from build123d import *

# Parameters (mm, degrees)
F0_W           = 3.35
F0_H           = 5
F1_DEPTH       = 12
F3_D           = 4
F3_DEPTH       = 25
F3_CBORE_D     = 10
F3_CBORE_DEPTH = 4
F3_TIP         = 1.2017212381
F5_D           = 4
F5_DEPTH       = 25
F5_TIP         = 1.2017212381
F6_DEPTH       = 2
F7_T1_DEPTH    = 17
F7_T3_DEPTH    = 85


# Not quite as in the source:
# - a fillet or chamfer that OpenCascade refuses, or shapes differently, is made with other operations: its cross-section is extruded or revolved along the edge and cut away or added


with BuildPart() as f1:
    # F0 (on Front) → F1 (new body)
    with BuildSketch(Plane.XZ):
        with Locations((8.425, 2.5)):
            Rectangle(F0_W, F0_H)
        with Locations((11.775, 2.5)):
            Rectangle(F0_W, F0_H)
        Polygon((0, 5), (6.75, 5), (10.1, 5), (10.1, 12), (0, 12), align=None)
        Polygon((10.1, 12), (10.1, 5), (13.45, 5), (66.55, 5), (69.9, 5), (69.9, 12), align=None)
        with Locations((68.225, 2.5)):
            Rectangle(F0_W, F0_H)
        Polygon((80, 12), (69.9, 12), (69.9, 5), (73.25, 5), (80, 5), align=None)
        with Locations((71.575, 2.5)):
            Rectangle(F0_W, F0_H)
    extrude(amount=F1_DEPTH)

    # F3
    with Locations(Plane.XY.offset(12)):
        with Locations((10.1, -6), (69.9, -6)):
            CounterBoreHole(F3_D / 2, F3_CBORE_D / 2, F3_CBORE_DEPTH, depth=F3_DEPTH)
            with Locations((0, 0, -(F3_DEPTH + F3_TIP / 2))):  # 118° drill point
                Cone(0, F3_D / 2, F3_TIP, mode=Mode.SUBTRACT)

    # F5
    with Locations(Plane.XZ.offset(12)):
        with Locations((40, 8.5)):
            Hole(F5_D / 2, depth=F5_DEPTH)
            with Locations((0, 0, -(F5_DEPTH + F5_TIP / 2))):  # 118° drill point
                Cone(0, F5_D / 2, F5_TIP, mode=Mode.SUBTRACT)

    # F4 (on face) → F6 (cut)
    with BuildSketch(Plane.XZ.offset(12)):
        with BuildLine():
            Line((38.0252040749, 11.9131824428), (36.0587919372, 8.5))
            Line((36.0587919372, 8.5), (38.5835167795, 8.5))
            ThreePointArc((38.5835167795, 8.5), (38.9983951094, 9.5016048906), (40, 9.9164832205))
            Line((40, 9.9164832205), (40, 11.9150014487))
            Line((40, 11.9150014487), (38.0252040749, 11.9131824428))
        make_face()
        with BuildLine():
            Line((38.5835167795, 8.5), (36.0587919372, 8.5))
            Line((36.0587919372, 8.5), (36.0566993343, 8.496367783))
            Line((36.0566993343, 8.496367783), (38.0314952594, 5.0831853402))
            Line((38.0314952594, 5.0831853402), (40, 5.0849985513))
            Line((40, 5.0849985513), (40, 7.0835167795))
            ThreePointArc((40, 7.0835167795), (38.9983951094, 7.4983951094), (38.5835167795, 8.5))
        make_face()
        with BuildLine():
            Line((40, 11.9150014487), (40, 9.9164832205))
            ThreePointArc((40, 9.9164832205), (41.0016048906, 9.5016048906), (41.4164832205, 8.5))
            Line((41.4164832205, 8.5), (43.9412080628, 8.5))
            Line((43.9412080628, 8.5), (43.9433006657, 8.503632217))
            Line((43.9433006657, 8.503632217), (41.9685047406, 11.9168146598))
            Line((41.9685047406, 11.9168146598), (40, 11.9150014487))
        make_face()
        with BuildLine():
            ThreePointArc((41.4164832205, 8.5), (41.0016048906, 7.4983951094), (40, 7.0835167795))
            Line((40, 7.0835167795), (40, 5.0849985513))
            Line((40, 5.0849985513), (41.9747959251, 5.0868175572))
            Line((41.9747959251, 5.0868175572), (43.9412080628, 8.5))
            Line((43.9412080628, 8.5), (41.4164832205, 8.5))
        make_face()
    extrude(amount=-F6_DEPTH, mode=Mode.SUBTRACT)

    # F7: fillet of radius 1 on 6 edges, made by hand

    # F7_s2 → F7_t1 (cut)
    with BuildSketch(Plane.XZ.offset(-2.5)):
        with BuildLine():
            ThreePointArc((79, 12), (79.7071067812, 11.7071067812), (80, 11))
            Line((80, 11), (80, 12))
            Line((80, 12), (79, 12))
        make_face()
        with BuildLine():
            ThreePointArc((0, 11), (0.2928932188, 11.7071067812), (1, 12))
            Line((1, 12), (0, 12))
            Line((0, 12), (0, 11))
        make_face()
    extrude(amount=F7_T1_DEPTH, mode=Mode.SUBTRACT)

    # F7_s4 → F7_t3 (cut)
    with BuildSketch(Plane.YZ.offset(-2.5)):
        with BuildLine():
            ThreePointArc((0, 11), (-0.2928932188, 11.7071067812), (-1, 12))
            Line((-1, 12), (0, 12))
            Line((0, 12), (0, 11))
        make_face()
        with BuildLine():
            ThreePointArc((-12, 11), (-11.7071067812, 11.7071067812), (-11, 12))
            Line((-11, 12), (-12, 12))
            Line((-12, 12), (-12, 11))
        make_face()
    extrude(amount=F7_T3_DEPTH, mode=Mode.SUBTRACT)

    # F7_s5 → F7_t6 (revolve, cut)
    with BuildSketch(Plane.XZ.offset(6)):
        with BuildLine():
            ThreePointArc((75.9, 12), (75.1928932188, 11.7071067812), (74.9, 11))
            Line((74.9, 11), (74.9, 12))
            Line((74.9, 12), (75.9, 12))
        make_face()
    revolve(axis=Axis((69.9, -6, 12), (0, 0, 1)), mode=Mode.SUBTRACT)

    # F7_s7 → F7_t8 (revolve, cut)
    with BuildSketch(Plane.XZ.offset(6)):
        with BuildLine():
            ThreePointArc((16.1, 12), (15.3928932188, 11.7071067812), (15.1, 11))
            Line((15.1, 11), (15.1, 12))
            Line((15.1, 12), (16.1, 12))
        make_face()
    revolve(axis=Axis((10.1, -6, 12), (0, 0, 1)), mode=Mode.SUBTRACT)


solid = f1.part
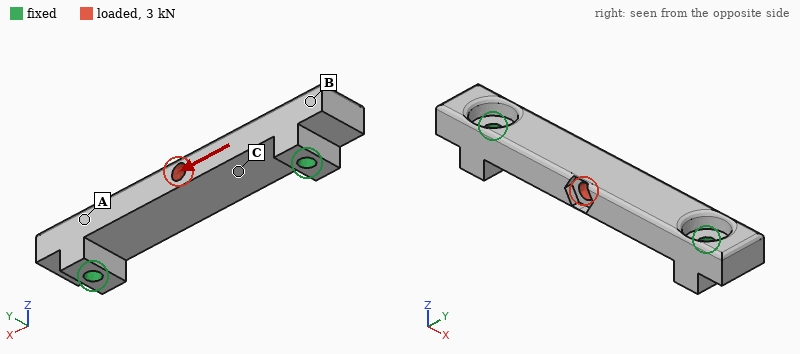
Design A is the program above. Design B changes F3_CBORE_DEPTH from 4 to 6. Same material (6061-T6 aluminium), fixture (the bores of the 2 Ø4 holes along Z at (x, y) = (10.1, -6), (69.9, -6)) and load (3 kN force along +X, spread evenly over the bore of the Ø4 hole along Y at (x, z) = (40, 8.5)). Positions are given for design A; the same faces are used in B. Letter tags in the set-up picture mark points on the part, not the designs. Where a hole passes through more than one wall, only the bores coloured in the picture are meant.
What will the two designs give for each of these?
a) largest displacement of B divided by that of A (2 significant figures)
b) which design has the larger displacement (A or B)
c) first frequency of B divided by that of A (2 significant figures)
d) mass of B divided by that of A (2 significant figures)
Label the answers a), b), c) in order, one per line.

a) 1.6
b) B
c) 0.93
d) 0.96
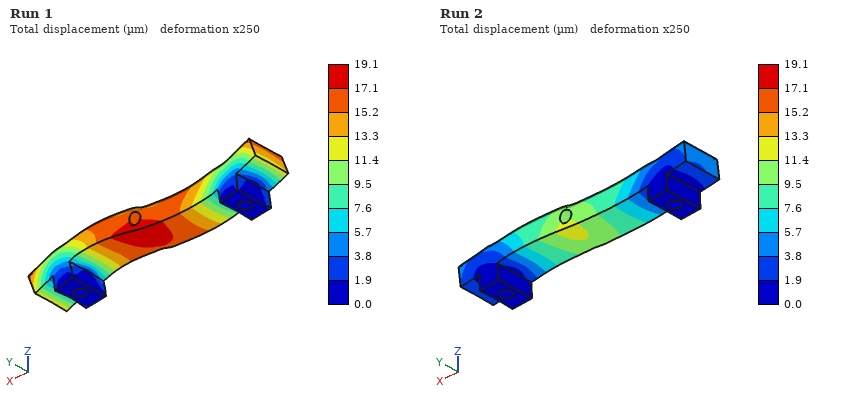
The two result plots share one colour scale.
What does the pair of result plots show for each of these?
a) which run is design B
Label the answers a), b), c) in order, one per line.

a) Run 1
